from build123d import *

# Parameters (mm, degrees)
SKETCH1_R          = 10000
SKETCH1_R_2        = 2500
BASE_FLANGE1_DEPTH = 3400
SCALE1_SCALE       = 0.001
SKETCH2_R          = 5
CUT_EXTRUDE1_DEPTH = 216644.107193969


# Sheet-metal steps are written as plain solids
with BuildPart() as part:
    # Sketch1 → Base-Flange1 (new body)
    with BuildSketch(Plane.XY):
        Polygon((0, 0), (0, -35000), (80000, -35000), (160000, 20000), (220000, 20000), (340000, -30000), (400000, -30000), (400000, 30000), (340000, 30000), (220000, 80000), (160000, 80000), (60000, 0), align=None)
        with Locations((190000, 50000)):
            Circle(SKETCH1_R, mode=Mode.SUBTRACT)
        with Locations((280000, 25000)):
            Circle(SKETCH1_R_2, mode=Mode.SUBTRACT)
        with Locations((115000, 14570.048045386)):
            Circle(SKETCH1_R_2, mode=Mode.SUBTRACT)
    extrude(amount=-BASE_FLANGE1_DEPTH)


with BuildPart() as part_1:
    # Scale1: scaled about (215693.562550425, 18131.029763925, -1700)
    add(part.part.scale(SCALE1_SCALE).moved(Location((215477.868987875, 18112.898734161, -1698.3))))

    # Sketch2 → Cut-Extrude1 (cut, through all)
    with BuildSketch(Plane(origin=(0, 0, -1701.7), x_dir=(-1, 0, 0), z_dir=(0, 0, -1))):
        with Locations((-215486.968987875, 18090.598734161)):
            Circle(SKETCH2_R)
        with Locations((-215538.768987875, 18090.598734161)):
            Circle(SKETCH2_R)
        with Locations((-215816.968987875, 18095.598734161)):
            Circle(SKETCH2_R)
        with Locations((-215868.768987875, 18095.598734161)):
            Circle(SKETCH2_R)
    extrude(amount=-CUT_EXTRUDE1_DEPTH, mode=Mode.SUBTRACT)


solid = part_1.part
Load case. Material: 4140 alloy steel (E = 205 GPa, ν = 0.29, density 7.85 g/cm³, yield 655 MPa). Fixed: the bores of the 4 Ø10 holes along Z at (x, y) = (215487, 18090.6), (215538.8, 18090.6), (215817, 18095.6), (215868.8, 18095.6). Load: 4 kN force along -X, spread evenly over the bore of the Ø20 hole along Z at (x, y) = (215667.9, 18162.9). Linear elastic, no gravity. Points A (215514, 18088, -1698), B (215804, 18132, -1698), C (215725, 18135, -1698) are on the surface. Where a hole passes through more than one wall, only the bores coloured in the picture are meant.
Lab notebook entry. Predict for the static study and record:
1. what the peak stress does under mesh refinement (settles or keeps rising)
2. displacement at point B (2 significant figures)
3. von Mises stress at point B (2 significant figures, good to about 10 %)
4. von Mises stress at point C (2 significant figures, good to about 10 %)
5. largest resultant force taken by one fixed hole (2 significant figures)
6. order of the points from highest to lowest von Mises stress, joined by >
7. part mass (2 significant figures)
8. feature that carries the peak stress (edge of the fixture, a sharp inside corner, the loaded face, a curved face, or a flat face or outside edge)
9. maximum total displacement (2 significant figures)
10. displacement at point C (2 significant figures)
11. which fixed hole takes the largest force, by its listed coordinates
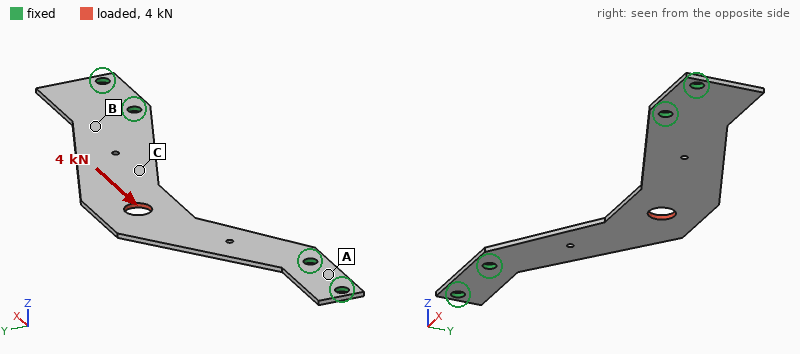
keeps rising
4.6 µm
12 MPa
18 MPa
1.7 kN
C > B > A
560 g
edge of the fixture
15 µm
10 µm
(215817, 18095.6)
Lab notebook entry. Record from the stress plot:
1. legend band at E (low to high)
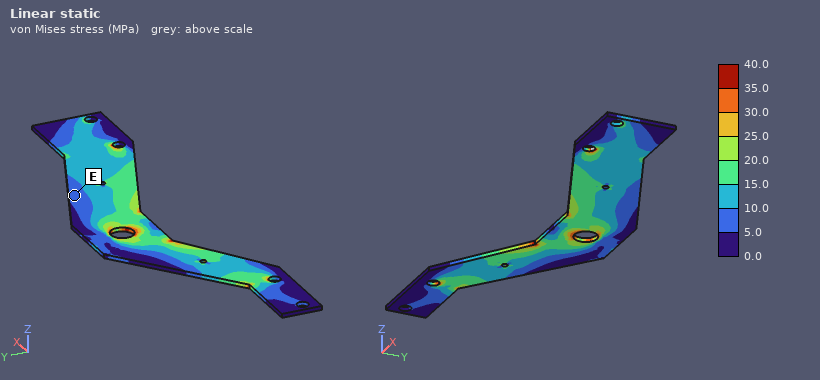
5.0 to 10.0 MPa
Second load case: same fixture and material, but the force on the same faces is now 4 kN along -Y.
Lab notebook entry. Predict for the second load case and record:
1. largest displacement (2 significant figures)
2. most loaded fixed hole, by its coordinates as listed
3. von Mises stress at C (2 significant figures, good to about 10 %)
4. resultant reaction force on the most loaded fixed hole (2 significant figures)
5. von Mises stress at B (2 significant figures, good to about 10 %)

40 µm
(215538.8, 18090.6)
16 MPa
3.5 kN
8.7 MPa
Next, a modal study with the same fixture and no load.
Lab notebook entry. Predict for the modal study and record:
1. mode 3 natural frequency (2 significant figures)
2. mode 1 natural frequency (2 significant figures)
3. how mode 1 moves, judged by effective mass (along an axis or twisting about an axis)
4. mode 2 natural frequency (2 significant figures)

650 Hz
150 Hz
along Z
460 Hz
